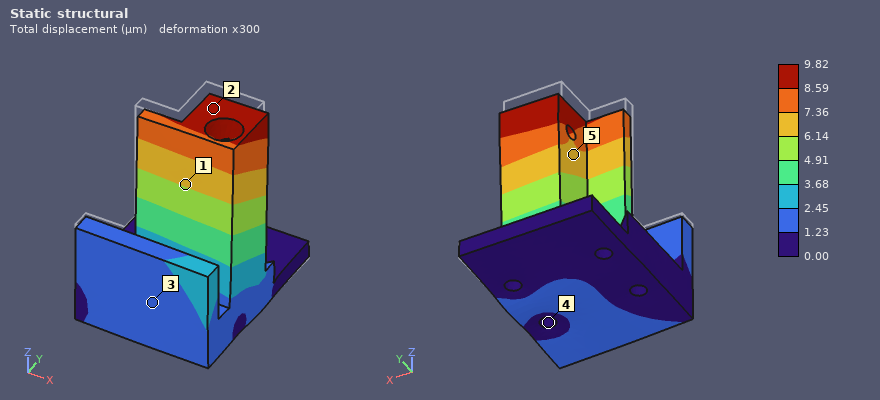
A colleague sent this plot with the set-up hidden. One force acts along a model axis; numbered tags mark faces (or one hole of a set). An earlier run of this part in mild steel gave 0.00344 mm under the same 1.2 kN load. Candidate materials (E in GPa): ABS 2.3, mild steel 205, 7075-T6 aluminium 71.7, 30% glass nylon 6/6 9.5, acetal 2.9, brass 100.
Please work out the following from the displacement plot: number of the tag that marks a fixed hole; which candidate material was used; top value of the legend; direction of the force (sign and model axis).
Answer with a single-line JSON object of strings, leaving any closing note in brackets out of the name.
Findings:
{"number of the tag that marks a fixed hole": "4", "which candidate material was used": "7075-T6 aluminium", "top value of the legend": "9.82 µm", "direction of the force": "-Z"}
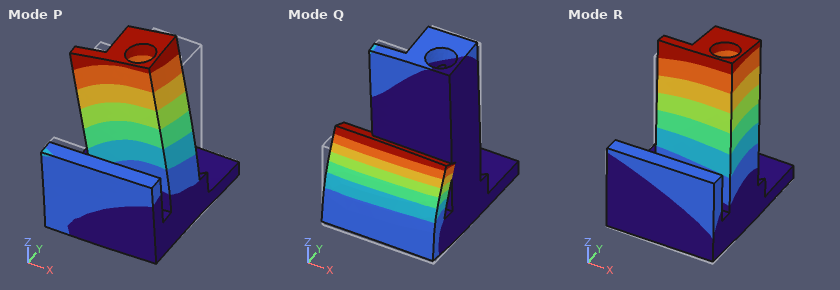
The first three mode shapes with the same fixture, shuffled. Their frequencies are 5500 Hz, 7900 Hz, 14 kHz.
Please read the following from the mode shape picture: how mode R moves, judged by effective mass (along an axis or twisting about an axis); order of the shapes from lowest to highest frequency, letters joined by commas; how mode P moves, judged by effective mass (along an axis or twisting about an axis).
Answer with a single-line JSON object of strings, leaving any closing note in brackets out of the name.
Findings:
{"how mode R moves, judged by effective mass": "along Y", "order of the shapes from lowest to highest frequency, letters joined by commas": "R, P, Q", "how mode P moves, judged by effective mass": "along X"}
